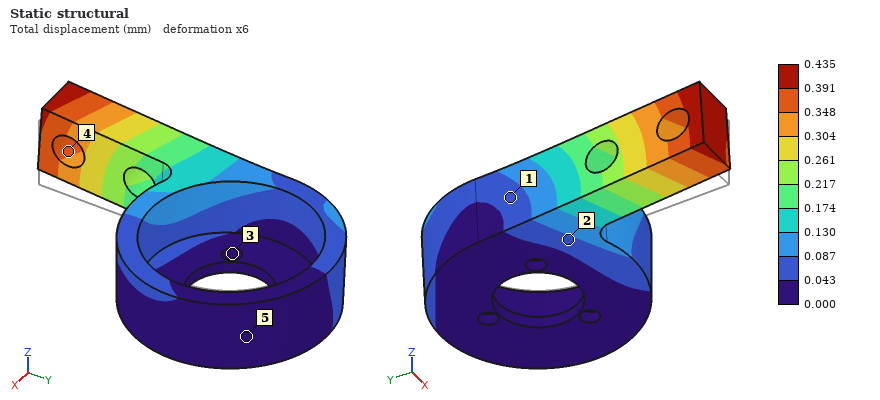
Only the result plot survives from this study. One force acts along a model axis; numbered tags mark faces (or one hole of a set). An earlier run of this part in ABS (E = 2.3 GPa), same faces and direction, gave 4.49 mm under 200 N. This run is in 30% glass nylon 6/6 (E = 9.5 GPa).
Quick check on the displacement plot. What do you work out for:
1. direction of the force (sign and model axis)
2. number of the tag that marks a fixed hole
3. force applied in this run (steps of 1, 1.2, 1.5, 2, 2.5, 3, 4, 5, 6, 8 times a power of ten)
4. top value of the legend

+Z
3
80 N
0.435 mm
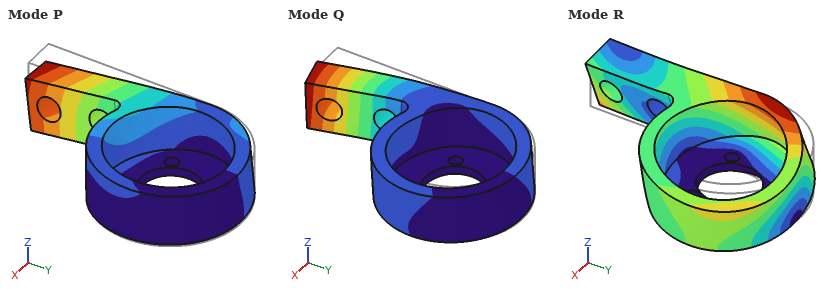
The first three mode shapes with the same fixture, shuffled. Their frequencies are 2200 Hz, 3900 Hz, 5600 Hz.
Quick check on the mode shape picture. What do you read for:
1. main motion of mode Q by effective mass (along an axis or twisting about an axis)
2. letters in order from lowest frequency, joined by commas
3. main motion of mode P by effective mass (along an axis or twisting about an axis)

along X
P, Q, R
along Z
